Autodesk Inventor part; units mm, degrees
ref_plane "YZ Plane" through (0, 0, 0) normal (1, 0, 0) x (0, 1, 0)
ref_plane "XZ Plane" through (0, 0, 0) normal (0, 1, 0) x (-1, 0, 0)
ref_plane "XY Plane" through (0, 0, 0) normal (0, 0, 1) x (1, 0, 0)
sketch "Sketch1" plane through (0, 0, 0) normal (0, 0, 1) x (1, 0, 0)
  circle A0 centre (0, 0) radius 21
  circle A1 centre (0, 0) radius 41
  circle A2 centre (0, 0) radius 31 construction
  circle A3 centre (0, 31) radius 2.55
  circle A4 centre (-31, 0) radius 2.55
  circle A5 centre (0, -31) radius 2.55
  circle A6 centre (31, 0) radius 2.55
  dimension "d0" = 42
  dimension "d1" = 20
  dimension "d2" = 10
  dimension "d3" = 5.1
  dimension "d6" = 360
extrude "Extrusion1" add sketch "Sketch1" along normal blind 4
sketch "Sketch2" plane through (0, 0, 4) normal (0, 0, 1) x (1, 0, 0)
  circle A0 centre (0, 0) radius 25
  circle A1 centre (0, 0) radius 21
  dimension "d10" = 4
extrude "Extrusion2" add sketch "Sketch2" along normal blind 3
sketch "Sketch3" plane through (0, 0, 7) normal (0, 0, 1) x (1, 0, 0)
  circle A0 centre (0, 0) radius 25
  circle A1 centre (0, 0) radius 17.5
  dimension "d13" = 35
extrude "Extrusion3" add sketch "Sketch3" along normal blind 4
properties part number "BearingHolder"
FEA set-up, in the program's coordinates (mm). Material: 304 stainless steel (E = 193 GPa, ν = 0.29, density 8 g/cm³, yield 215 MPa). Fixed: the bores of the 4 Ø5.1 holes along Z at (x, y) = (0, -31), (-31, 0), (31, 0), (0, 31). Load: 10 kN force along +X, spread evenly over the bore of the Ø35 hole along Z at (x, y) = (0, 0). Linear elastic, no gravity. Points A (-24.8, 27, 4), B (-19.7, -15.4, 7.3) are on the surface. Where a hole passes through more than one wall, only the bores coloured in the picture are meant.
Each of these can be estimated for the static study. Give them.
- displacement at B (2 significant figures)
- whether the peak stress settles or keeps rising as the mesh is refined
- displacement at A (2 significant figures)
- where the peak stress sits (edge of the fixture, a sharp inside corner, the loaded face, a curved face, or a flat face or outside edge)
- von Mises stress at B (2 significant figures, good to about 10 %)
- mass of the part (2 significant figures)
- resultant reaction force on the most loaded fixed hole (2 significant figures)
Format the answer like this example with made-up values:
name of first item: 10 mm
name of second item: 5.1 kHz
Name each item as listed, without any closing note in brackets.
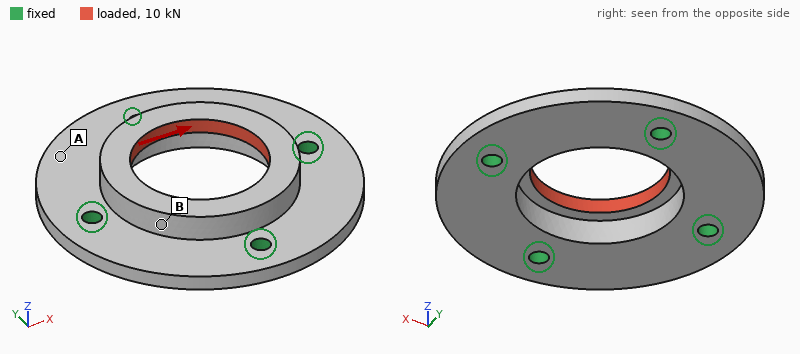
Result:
displacement at B: 7.4 µm
whether the peak stress settles or keeps rising as the mesh is refined: keeps rising
displacement at A: 8.2 µm
where the peak stress sits: edge of the fixture
von Mises stress at B: 30 MPa
mass of the part: 170 g
resultant reaction force on the most loaded fixed hole: 2.7 kN
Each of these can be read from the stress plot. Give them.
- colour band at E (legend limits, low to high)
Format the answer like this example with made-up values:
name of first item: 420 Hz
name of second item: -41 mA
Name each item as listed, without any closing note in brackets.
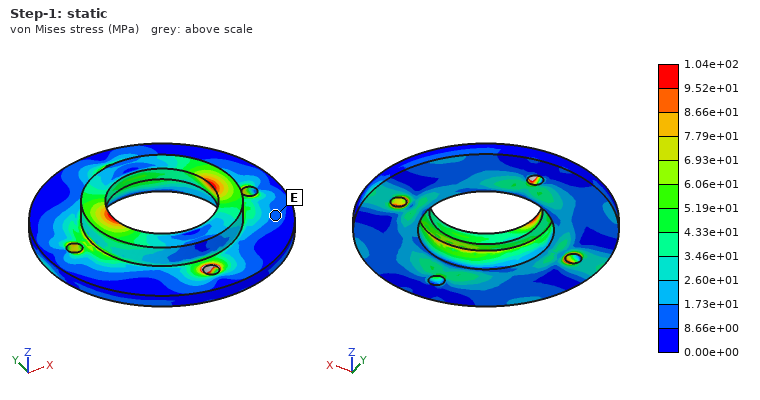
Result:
colour band at E: 8.66e+00 to 1.73e+01 MPa
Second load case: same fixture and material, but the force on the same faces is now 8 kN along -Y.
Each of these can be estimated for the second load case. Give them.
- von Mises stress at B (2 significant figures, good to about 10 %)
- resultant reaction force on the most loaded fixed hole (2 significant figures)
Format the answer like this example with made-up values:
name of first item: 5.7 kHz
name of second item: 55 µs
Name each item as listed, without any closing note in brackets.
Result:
von Mises stress at B: 19 MPa
resultant reaction force on the most loaded fixed hole: 2.2 kN
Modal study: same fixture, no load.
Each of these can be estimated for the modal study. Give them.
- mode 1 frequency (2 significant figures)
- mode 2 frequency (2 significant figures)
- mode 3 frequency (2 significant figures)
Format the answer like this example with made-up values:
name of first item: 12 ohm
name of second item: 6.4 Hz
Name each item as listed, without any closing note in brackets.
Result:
mode 1 frequency: 7700 Hz
mode 2 frequency: 8700 Hz
mode 3 frequency: 8700 Hz
